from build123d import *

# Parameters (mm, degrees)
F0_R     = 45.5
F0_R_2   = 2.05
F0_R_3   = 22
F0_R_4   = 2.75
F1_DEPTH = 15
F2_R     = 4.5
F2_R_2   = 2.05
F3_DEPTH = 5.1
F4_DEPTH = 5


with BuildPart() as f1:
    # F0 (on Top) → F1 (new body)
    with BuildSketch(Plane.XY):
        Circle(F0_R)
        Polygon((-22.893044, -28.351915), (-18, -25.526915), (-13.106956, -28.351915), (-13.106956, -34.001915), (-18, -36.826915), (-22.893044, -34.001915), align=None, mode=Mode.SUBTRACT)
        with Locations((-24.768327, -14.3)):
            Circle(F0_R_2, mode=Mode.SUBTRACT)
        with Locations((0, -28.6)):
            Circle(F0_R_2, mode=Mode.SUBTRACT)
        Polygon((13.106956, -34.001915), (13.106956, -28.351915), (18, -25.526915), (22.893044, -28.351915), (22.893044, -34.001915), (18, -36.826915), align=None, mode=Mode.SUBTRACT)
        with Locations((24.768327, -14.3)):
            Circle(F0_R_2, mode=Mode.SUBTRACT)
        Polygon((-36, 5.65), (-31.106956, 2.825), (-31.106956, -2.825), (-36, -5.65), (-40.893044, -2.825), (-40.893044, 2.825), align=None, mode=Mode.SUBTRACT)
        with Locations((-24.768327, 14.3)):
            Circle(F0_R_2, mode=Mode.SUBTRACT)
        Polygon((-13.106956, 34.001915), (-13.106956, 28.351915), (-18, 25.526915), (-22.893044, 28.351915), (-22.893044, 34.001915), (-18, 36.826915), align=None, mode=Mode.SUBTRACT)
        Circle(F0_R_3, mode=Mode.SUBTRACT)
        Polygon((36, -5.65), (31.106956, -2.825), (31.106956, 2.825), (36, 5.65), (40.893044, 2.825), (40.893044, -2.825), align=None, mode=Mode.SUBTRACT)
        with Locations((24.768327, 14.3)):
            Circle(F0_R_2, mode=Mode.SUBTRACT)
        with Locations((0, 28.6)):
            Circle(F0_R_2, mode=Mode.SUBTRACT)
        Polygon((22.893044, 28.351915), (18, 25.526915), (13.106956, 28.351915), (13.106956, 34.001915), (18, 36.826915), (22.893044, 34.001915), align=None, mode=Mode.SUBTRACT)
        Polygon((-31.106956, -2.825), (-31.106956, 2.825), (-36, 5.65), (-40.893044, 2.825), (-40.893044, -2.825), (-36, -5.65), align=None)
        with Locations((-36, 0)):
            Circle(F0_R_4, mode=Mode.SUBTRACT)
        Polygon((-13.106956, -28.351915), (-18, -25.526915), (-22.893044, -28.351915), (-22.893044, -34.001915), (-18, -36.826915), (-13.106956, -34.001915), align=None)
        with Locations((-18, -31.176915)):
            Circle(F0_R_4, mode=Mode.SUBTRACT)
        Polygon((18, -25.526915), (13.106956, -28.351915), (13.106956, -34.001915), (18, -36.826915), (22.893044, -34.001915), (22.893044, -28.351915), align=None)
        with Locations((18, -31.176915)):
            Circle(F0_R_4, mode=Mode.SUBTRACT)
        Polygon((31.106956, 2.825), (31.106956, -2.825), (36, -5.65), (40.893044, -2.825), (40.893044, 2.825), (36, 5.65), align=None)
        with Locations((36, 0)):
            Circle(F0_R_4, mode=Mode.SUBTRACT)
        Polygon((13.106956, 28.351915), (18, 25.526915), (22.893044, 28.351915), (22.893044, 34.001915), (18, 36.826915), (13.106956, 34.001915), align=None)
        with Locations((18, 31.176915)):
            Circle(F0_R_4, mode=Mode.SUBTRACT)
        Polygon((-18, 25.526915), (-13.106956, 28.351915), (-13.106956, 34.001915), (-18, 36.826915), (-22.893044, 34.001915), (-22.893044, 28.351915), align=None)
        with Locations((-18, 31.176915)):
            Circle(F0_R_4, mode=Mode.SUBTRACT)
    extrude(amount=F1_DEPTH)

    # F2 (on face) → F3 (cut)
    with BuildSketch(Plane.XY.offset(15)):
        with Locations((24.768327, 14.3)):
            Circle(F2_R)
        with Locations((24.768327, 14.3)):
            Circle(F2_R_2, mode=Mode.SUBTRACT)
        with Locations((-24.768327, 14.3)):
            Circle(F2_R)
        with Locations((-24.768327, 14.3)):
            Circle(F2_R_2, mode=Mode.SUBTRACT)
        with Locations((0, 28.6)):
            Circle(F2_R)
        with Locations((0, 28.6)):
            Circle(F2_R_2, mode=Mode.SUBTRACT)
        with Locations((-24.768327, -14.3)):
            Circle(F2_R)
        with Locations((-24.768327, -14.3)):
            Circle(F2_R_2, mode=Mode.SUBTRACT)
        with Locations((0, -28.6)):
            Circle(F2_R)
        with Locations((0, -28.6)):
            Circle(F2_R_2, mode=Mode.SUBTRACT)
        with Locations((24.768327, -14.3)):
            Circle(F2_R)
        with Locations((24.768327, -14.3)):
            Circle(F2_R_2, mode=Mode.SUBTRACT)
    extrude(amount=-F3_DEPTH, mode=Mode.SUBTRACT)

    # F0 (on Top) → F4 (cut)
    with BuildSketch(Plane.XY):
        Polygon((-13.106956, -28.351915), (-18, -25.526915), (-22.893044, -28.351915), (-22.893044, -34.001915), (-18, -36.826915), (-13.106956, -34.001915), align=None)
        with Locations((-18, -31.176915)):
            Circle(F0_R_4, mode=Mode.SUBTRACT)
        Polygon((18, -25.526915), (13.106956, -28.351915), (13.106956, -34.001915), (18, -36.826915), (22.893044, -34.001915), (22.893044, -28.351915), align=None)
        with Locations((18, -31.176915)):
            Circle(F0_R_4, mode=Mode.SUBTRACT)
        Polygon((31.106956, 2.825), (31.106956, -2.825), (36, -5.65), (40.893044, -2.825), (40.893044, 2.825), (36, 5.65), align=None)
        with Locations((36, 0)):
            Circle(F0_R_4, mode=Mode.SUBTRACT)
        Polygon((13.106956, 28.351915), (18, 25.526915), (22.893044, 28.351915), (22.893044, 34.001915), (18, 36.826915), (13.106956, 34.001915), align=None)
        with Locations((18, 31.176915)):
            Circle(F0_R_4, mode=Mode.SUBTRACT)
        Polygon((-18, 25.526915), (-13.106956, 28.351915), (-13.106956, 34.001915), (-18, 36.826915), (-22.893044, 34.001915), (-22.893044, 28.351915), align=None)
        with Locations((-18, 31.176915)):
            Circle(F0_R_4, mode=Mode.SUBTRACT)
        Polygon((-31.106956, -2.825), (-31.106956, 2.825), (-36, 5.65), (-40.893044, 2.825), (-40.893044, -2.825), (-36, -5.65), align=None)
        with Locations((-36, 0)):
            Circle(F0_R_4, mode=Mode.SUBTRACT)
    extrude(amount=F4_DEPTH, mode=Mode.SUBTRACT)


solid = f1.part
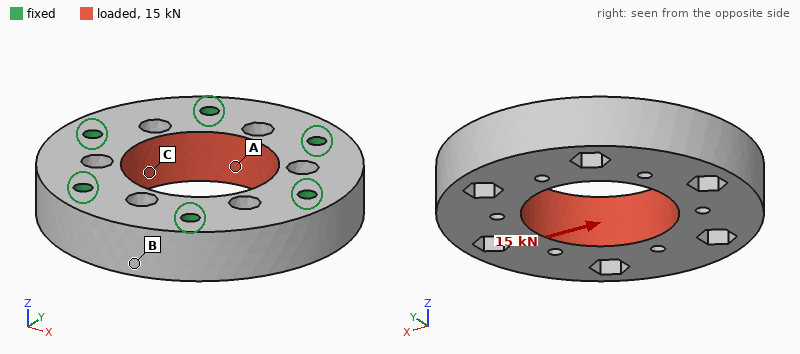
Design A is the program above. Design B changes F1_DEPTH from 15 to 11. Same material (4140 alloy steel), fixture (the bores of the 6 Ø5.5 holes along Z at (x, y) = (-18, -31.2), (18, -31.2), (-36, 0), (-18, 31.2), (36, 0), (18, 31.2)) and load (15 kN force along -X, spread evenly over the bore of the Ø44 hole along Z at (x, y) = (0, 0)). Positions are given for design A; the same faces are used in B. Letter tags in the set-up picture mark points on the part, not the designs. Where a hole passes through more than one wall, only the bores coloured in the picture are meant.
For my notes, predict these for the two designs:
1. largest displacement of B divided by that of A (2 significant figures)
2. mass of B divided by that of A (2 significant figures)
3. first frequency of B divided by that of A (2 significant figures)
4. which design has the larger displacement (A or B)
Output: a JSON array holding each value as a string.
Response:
["1.6", "0.74", "0.80", "B"]
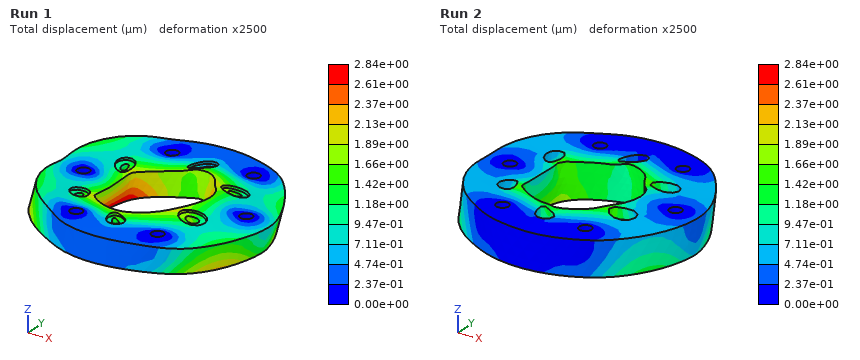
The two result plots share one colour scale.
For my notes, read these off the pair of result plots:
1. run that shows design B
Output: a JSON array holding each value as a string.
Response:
["Run 1"]
